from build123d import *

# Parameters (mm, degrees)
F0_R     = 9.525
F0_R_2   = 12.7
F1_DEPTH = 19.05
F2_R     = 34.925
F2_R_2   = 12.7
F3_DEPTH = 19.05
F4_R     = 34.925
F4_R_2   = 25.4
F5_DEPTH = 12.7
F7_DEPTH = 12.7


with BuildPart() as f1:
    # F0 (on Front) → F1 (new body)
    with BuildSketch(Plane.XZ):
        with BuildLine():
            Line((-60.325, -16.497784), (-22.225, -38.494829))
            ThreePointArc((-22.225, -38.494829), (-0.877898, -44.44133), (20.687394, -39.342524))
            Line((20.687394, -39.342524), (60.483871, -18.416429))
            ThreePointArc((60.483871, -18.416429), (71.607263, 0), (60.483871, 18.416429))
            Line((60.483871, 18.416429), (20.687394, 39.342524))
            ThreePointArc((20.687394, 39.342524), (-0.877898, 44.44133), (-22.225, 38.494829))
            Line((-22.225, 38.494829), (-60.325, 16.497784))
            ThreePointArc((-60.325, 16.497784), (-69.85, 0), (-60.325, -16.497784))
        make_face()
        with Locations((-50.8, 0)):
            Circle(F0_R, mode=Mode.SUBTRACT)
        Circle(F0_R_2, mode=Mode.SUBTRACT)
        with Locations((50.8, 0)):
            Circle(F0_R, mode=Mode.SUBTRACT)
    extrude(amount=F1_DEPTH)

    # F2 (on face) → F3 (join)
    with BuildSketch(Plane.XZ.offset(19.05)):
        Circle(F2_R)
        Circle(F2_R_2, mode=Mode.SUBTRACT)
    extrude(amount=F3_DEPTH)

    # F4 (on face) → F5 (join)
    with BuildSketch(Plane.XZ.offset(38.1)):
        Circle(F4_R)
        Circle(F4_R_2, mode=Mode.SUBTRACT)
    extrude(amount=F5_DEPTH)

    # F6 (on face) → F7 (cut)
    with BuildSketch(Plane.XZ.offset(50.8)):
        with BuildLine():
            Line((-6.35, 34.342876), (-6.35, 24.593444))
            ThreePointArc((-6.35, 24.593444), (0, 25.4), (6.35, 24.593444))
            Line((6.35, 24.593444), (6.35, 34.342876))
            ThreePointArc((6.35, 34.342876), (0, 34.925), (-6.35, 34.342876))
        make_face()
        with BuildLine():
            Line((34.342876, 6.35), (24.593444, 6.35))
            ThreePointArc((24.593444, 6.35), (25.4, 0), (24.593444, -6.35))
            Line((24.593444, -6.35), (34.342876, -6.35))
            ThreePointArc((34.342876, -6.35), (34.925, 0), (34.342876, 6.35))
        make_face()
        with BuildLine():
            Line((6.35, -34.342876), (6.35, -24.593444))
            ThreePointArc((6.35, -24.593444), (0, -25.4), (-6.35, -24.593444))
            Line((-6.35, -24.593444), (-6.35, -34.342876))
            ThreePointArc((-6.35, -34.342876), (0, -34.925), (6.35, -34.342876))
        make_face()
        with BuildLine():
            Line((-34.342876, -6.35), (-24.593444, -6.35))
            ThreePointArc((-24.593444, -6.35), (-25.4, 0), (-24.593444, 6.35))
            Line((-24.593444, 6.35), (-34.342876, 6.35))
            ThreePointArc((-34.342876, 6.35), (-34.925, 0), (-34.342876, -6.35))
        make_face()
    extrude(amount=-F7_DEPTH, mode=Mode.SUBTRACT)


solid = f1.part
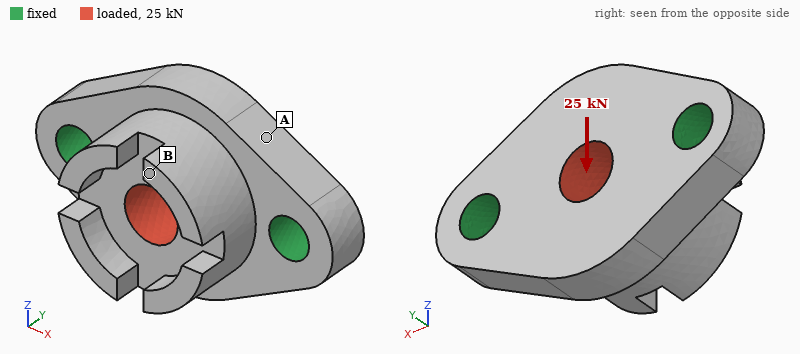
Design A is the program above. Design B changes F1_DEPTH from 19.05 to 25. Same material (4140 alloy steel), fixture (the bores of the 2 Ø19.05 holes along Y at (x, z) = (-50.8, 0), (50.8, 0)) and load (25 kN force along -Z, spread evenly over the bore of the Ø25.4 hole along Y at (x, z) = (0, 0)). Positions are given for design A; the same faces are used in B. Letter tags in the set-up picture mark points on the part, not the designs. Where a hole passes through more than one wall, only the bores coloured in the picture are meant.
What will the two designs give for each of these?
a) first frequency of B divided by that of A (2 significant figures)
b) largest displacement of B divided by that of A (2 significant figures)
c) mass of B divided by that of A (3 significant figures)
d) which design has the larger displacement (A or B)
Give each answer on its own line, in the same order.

1.3
0.48
1.11
A
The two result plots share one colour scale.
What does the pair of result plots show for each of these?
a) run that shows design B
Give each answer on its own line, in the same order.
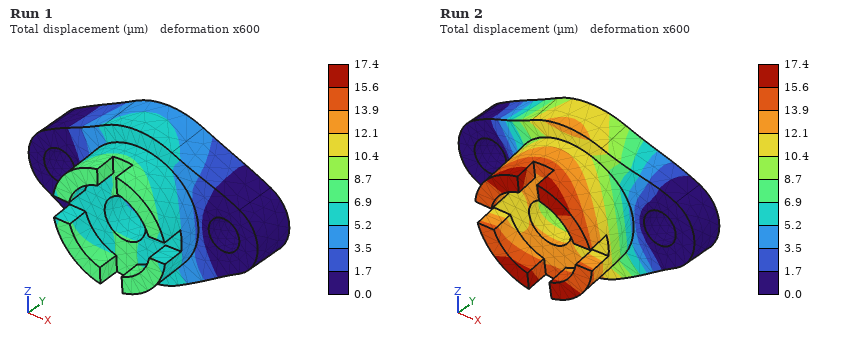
Run 1
